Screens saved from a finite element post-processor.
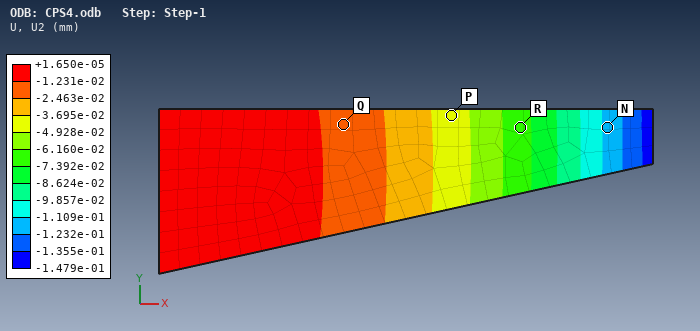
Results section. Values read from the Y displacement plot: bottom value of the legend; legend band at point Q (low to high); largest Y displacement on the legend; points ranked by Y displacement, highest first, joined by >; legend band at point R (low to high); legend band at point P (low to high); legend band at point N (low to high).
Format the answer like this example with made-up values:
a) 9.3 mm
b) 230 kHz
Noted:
a) -1.479e-01 mm
b) -2.463e-02 to -1.231e-02 mm
c) +1.650e-05 mm
d) Q > P > R > N
e) -7.392e-02 to -6.160e-02 mm
f) -4.928e-02 to -3.695e-02 mm
g) -1.232e-01 to -1.109e-01 mm
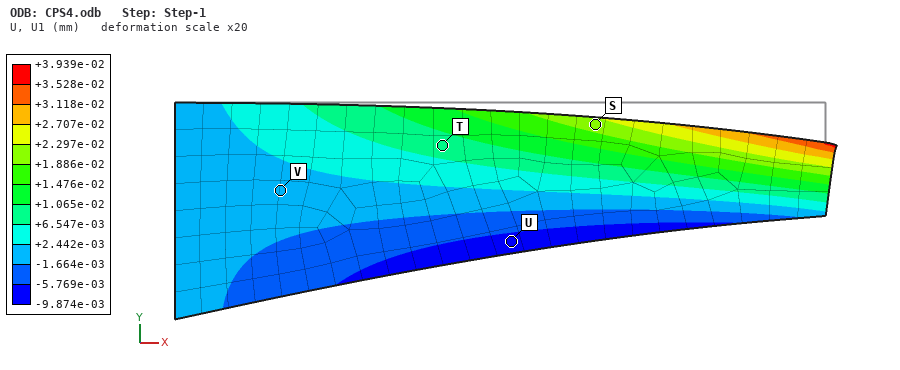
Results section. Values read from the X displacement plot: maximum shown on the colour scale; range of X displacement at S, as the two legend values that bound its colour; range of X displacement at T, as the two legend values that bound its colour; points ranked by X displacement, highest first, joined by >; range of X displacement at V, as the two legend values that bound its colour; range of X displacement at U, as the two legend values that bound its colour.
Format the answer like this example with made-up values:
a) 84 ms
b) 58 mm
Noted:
a) +3.939e-02 mm
b) +1.886e-02 to +2.297e-02 mm
c) +6.547e-03 to +1.065e-02 mm
d) S > T > V > U
e) -1.664e-03 to +2.442e-03 mm
f) -9.874e-03 to -5.769e-03 mm
